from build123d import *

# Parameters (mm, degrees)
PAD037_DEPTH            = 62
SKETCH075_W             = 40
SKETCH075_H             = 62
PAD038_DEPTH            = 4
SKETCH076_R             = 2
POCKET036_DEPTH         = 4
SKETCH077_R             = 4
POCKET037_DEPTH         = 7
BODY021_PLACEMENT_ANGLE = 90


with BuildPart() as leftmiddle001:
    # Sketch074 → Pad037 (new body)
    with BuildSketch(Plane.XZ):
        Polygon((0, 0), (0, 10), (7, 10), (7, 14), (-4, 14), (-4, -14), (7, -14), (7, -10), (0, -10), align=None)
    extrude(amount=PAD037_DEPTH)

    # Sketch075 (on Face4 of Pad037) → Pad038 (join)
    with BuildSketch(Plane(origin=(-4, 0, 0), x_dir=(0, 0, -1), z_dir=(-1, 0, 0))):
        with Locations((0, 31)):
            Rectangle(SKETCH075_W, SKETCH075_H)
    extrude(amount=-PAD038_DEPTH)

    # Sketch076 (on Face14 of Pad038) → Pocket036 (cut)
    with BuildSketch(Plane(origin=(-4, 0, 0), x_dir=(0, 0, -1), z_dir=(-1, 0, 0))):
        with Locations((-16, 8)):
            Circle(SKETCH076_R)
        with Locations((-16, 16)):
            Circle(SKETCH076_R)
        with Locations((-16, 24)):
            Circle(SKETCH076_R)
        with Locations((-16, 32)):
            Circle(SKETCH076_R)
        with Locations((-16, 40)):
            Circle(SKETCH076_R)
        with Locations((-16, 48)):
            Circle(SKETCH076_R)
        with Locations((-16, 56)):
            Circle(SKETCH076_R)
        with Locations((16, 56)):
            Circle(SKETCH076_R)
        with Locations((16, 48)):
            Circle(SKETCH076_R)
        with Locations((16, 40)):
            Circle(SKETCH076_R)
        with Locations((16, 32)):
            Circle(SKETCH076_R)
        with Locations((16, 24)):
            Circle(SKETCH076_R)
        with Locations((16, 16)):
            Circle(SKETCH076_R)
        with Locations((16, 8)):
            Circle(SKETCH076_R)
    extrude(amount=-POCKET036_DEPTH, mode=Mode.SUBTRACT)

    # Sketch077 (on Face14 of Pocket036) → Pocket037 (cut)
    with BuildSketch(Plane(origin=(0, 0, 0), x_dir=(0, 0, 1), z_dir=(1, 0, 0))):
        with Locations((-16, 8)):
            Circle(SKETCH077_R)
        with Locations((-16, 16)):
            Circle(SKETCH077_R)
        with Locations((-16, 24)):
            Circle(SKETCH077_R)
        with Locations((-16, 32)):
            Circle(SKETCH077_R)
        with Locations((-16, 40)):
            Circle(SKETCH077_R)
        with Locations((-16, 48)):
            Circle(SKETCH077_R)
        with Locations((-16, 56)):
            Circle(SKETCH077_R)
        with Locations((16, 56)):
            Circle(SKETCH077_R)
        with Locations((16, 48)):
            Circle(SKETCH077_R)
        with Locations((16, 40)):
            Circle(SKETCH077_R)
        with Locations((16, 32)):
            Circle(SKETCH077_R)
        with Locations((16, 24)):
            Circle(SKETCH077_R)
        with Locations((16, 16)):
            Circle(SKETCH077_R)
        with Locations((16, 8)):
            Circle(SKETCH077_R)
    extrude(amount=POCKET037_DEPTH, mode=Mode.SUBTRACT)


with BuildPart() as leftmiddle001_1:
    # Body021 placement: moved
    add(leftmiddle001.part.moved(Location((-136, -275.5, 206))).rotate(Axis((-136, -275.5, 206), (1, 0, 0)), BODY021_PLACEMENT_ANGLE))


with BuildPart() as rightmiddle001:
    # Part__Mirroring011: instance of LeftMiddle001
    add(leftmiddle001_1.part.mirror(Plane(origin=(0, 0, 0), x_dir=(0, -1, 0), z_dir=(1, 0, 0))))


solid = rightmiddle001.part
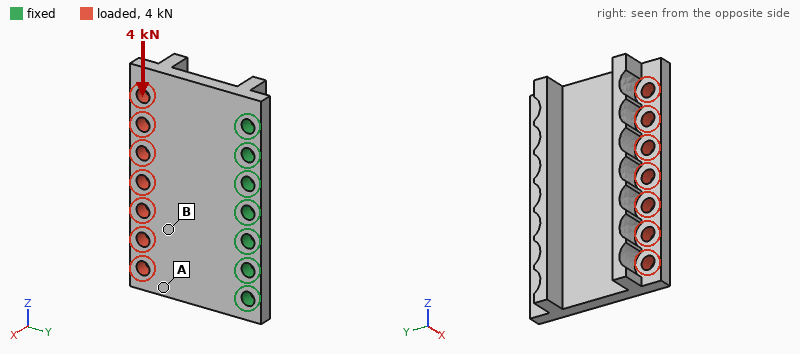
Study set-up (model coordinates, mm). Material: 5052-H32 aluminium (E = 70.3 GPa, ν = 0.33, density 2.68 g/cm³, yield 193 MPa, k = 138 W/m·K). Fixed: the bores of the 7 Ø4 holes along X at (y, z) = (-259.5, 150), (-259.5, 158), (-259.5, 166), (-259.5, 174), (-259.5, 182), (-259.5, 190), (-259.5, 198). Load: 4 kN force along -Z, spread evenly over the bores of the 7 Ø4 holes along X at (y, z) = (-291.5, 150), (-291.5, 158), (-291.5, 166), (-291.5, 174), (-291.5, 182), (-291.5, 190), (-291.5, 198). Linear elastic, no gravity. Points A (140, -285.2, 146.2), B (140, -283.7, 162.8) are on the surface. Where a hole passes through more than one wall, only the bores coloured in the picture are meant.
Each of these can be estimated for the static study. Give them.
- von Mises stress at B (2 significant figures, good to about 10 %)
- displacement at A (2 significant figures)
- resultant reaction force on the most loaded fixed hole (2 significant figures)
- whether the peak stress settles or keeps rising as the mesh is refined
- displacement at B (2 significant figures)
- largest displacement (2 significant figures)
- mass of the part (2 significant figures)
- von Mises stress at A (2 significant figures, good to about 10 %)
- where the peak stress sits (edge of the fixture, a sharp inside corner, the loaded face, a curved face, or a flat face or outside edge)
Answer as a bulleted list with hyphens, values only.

- 37 MPa
- 28 µm
- 2.1 kN
- keeps rising
- 22 µm
- 42 µm
- 31 g
- 13 MPa
- edge of the fixture
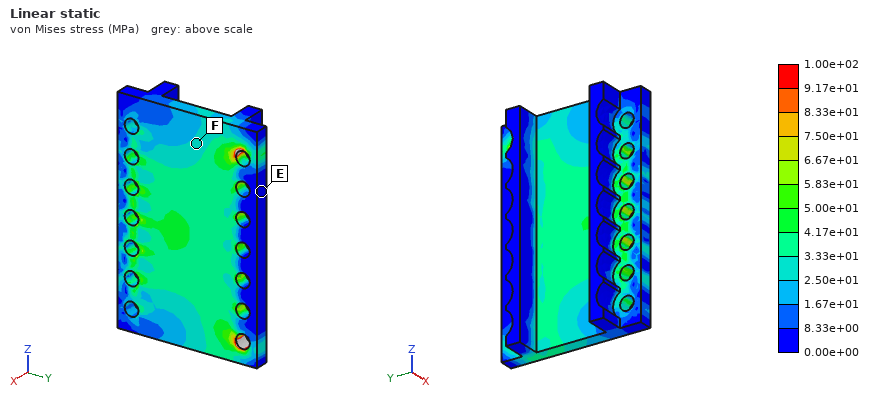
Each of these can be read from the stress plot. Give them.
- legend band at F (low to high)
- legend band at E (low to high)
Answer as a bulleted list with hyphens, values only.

- 2.50e+01 to 3.33e+01 MPa
- 0.00e+00 to 8.33e+00 MPa
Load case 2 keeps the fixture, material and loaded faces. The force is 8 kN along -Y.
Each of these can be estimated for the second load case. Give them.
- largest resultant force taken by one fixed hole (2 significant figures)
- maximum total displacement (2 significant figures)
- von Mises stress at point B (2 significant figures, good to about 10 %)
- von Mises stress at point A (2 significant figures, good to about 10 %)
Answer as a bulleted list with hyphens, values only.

- 1.5 kN
- 20 µm
- 37 MPa
- 28 MPa
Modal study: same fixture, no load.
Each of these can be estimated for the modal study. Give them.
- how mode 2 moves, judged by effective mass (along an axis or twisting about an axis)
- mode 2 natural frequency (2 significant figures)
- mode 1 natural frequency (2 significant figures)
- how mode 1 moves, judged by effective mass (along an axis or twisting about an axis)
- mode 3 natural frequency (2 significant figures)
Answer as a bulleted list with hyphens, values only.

- twisting about Y
- 4100 Hz
- 2700 Hz
- along X
- 12 kHz
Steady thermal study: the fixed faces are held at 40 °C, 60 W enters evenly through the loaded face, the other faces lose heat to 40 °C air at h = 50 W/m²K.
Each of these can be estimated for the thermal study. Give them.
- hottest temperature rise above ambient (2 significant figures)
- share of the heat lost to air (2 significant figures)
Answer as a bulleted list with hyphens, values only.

- 54 K
- 14 %
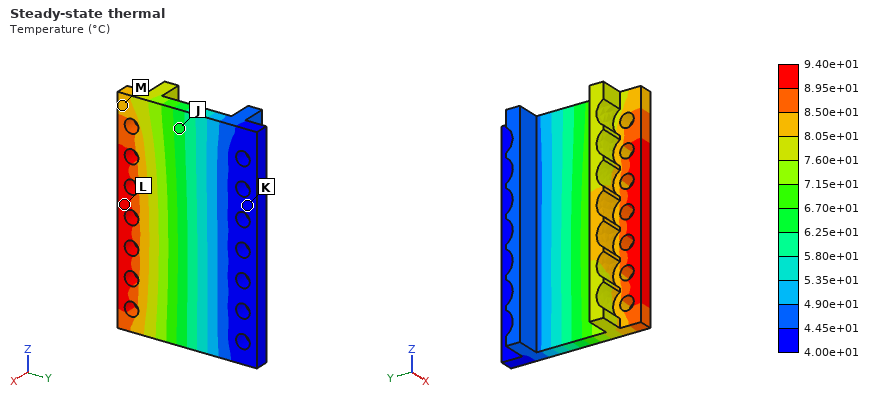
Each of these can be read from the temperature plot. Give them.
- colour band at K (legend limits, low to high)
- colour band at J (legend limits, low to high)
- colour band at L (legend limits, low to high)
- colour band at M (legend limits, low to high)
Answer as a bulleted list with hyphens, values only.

- 4.00e+01 to 4.45e+01 °C
- 6.25e+01 to 6.70e+01 °C
- 8.95e+01 to 9.40e+01 °C
- 8.05e+01 to 8.50e+01 °C
